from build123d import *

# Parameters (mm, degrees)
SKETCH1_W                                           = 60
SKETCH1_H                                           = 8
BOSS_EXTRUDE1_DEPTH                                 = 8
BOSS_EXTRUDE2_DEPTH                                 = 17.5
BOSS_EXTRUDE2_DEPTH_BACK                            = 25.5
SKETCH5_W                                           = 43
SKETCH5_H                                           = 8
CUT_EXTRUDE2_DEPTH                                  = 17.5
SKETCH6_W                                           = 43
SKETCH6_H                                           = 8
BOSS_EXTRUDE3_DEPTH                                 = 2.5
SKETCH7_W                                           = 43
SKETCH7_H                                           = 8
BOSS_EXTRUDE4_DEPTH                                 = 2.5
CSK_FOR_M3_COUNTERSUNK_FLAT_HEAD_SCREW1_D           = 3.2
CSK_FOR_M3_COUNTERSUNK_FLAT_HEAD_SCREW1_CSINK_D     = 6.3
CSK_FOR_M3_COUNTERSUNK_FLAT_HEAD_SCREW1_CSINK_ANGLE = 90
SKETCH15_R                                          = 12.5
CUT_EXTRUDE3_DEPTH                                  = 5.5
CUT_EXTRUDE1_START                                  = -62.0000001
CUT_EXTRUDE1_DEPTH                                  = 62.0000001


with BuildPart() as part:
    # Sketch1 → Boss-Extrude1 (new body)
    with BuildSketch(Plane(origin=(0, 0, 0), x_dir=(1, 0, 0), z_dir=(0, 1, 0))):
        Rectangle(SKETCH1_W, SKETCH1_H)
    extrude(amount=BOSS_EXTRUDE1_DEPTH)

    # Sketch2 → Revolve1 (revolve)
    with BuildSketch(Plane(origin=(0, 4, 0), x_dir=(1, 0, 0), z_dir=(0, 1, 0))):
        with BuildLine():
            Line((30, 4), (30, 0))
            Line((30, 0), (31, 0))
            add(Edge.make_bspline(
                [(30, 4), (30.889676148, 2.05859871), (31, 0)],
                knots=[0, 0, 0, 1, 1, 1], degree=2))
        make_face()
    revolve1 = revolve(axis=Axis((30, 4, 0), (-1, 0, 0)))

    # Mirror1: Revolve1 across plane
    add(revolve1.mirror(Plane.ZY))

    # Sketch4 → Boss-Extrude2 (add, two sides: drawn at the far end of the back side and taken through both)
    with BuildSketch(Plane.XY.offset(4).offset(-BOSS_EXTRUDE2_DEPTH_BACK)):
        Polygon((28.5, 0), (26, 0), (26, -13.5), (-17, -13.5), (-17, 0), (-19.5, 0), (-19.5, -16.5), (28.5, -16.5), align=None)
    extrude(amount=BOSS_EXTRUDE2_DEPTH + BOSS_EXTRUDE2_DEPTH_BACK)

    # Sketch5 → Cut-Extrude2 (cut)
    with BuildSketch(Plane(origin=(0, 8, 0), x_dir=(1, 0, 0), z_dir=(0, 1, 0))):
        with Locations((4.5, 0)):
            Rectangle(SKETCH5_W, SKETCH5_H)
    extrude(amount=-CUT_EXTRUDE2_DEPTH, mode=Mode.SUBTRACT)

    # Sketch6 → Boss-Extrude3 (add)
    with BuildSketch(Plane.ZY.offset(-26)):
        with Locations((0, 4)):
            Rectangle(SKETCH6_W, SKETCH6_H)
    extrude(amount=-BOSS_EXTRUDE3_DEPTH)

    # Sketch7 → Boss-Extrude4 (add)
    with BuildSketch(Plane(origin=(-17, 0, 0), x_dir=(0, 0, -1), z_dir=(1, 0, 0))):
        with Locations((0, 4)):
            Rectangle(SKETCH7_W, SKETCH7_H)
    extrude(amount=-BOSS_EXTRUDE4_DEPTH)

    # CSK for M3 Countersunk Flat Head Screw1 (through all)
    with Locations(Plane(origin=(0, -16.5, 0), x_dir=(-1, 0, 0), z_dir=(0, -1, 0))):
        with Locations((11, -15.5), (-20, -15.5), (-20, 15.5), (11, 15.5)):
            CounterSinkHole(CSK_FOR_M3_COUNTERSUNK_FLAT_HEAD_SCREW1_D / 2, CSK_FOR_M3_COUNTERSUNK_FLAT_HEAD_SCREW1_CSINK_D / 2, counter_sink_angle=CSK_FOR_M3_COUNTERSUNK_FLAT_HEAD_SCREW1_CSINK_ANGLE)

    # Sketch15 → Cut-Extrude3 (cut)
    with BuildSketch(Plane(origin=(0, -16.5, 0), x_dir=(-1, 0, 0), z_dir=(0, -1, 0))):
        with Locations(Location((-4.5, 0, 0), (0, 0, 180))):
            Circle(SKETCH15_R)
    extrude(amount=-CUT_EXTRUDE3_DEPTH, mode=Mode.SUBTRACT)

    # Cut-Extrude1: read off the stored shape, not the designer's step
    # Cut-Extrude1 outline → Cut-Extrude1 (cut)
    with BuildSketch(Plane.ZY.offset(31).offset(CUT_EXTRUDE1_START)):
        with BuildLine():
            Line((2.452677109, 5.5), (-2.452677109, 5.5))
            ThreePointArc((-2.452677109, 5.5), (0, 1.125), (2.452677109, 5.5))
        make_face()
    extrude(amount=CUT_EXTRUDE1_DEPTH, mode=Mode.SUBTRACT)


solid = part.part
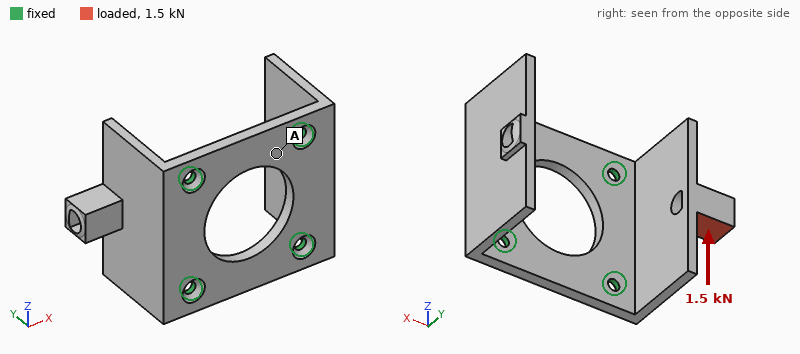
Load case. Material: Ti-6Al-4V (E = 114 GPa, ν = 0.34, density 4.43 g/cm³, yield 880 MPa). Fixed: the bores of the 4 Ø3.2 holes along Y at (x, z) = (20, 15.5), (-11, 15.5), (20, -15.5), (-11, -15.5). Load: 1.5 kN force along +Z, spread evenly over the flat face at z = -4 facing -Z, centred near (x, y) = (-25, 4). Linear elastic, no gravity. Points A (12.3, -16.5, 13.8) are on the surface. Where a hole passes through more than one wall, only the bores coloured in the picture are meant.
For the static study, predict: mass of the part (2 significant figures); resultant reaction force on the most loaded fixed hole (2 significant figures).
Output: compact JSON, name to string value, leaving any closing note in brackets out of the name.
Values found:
{"mass of the part": "43 g", "resultant reaction force on the most loaded fixed hole": "1.3 kN"}
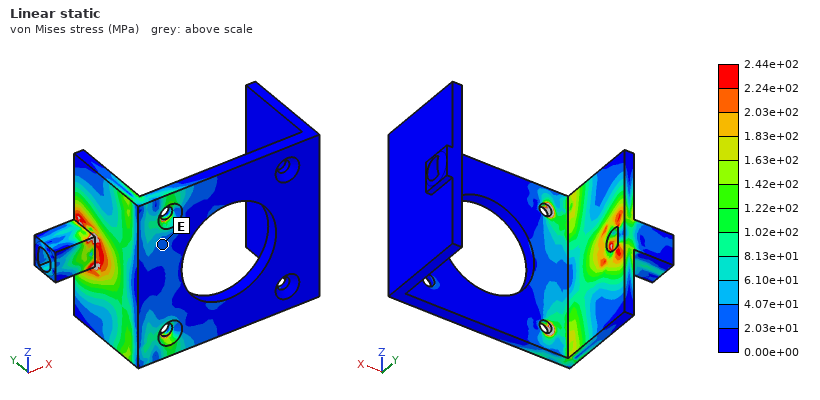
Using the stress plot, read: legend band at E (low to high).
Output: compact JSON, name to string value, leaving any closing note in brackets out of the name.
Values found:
{"legend band at E": "2.03e+01 to 4.07e+01 MPa"}
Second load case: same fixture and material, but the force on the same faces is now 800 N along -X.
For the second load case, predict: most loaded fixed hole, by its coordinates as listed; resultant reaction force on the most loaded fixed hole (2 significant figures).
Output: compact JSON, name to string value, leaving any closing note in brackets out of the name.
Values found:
{"most loaded fixed hole, by its coordinates as listed": "(-11, -15.5)", "resultant reaction force on the most loaded fixed hole": "900 N"}
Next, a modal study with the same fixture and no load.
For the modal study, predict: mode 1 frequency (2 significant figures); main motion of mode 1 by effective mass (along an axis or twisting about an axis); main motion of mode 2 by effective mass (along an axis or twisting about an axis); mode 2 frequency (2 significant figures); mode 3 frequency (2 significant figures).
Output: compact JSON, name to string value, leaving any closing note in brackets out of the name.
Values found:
{"mode 1 frequency": "2200 Hz", "main motion of mode 1 by effective mass": "along X", "main motion of mode 2 by effective mass": "along X", "mode 2 frequency": "2700 Hz", "mode 3 frequency": "5100 Hz"}
